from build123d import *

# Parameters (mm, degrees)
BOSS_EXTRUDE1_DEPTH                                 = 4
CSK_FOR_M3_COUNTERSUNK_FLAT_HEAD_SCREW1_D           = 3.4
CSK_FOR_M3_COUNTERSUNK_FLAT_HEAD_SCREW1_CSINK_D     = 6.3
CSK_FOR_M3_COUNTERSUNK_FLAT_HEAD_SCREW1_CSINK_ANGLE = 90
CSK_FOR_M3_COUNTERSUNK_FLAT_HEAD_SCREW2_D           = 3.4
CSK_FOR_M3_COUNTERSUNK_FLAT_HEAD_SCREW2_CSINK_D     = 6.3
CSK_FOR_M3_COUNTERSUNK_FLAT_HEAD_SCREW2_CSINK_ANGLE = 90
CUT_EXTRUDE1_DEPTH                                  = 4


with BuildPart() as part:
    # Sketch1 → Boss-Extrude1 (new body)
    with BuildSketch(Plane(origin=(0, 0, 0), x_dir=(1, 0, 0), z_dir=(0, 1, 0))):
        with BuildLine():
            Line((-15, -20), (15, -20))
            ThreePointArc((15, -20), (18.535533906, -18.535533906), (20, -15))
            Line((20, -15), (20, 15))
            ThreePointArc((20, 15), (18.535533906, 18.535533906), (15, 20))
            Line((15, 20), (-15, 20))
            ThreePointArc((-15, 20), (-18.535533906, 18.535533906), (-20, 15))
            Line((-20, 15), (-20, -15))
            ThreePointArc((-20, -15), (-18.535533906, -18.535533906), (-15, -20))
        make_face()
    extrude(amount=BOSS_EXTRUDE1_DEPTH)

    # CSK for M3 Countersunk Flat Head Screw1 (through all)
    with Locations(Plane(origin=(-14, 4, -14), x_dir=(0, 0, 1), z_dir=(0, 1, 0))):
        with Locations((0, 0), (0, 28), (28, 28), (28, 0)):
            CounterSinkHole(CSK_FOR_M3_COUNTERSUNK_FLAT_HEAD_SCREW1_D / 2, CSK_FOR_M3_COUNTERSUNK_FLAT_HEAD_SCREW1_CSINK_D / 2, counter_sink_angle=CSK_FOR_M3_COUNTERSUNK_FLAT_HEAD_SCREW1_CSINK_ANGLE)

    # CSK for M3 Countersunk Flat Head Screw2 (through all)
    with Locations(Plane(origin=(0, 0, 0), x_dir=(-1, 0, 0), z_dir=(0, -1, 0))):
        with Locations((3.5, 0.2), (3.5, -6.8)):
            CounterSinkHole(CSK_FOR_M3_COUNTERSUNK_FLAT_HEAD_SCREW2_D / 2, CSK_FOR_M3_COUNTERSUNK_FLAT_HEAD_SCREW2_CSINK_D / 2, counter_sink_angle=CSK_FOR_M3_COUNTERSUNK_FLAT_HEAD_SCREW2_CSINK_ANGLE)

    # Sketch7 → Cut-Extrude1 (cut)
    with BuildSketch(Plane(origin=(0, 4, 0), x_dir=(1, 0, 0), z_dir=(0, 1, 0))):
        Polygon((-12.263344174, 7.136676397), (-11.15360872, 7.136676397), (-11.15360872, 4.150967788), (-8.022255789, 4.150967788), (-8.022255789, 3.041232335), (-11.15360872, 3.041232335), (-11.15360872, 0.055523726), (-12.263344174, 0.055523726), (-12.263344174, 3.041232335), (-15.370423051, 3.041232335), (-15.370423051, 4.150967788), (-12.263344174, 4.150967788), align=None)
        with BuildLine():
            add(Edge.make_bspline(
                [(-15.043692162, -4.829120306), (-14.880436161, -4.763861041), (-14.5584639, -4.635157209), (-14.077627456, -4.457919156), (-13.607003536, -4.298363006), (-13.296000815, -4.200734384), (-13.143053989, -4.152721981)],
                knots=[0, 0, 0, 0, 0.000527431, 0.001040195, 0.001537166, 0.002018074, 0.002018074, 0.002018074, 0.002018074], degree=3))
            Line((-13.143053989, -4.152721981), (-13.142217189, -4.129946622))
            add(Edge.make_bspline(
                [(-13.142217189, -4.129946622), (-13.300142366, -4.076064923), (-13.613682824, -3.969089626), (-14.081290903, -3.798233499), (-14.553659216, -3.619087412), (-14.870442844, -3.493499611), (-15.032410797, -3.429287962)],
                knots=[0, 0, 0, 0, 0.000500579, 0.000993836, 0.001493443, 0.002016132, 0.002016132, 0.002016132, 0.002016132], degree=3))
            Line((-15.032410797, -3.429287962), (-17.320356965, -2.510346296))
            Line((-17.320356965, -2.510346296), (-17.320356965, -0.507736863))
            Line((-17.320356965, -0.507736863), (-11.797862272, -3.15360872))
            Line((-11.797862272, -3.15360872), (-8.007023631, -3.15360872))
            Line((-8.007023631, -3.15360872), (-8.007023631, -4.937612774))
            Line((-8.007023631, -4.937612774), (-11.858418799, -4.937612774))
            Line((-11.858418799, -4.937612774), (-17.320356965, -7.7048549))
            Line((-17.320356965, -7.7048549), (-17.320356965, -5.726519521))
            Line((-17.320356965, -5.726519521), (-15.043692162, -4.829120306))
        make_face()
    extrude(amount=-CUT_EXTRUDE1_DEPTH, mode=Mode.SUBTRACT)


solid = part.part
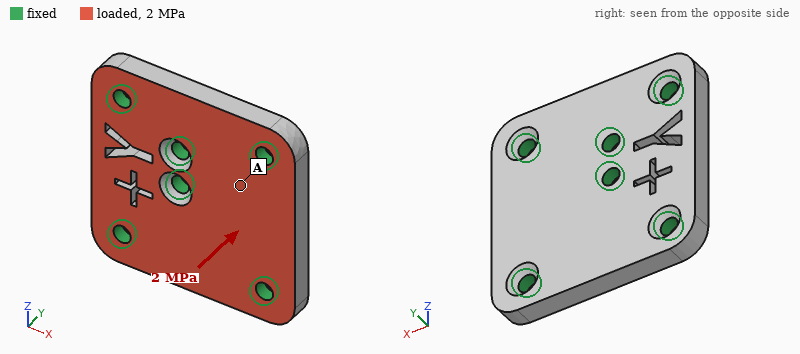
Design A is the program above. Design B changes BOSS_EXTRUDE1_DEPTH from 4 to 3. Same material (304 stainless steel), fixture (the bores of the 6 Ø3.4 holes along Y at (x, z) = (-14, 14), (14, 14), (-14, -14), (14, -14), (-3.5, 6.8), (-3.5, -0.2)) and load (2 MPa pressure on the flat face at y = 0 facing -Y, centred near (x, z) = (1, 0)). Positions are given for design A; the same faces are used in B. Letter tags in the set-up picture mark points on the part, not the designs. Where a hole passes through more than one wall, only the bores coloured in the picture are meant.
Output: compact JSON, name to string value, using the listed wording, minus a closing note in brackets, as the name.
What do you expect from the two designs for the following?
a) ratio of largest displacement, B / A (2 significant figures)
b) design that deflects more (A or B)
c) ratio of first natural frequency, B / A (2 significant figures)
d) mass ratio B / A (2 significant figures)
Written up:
{"ratio of largest displacement, B / A": "1.8", "design that deflects more": "B", "ratio of first natural frequency, B / A": "0.90", "mass ratio B / A": "0.76"}
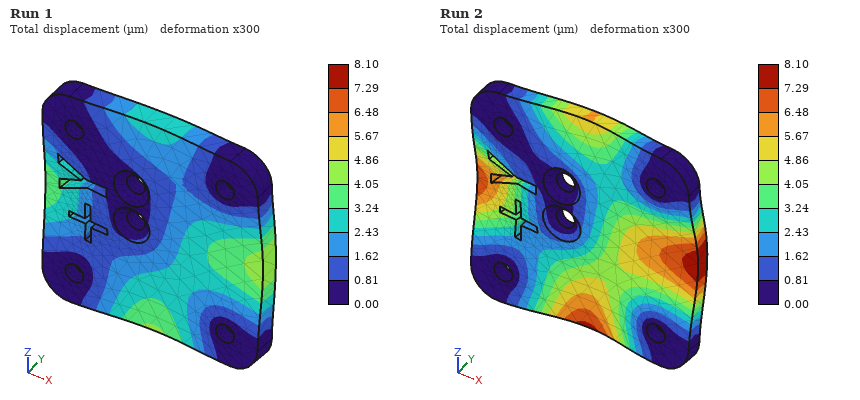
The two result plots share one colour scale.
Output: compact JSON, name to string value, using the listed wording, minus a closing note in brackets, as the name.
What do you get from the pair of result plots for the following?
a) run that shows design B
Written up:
{"run that shows design B": "Run 2"}
